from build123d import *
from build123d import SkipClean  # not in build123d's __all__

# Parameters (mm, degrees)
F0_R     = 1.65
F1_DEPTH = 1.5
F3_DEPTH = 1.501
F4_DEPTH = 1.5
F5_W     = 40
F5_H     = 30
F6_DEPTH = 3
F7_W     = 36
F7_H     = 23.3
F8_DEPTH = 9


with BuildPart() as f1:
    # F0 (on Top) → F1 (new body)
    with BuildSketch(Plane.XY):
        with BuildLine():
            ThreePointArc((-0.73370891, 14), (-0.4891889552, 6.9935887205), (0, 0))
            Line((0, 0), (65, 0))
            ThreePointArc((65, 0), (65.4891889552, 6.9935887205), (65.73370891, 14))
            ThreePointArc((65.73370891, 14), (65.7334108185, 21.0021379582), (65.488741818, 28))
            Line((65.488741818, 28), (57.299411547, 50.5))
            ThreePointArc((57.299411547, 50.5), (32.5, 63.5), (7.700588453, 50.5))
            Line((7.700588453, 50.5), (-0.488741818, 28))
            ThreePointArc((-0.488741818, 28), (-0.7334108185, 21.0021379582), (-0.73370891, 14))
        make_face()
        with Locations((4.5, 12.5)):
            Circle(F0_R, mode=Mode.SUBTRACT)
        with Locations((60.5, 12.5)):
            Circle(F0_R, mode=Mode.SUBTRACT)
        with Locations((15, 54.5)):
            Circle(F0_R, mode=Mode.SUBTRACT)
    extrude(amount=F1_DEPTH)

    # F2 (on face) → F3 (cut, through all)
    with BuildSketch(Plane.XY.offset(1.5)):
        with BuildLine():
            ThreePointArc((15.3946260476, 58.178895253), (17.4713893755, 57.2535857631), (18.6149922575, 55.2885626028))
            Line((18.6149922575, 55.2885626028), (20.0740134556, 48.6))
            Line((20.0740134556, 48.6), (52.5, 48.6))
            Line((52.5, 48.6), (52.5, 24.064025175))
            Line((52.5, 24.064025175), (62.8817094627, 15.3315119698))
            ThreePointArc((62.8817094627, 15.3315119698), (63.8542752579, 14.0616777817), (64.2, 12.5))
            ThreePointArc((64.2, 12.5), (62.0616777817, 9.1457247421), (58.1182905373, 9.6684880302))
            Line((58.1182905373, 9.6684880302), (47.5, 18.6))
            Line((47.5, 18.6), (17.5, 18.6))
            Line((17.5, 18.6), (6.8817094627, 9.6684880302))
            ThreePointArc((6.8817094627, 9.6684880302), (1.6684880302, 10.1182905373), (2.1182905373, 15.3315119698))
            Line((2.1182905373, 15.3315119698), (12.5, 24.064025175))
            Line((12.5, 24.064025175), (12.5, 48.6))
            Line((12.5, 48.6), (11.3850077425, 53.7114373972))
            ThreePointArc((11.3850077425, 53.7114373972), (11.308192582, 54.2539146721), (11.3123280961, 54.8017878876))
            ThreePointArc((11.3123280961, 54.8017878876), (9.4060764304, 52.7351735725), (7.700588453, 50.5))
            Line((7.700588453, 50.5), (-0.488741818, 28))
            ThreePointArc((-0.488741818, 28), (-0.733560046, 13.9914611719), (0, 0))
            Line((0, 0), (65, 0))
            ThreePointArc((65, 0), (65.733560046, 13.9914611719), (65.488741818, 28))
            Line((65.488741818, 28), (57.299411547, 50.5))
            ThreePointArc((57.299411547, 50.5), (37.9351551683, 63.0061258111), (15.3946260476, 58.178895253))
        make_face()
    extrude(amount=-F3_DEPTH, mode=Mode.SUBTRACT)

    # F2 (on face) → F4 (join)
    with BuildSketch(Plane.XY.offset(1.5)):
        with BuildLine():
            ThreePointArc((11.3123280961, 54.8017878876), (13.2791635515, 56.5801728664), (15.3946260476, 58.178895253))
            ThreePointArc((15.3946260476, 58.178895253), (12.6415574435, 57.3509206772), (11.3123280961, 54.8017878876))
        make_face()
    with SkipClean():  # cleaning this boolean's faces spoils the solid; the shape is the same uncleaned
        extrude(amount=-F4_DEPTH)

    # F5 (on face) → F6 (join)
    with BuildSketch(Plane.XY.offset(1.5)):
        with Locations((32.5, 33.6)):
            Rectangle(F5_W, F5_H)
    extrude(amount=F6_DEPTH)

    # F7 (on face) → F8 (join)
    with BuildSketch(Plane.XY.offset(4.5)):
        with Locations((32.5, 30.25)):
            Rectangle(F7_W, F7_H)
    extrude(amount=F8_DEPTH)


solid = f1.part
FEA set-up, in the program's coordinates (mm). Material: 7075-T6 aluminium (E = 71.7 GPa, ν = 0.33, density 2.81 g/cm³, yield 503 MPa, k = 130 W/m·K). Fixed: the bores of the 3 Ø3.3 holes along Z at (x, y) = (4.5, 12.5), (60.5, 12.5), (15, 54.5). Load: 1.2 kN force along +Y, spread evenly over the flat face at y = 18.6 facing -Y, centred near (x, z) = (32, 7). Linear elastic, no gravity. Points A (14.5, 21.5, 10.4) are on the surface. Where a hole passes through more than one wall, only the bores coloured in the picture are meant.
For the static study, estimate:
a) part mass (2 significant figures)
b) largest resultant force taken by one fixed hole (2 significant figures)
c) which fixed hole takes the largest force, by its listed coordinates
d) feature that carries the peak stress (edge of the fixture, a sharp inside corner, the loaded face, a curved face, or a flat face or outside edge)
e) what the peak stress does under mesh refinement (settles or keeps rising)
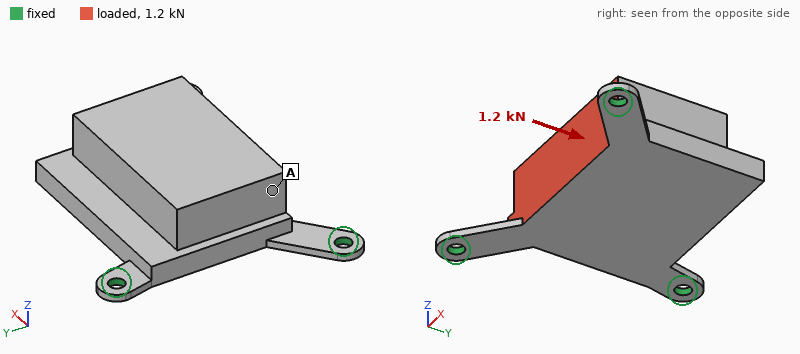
37 g
650 N
(15, 54.5)
edge of the fixture
keeps rising
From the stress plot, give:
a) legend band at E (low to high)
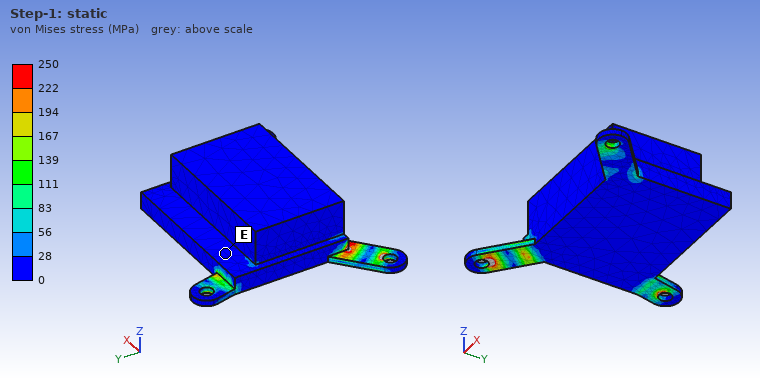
0 to 28 MPa
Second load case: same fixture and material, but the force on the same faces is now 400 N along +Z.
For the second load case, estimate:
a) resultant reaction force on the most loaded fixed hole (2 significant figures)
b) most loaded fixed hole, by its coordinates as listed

220 N
(60.5, 12.5)
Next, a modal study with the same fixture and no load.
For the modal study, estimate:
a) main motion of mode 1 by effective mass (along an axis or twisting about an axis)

along Z
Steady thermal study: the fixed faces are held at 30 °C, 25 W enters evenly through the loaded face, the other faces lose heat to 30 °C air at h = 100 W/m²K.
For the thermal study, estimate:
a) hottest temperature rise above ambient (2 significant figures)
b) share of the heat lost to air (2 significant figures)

37 K
48 %
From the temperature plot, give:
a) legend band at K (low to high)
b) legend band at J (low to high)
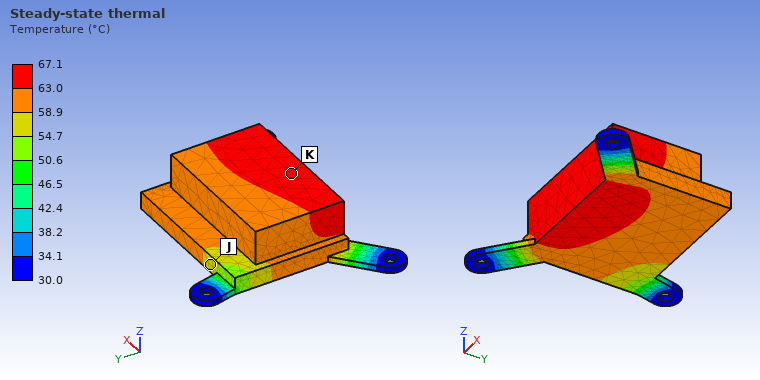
63.0 to 67.1 °C
54.7 to 58.9 °C
